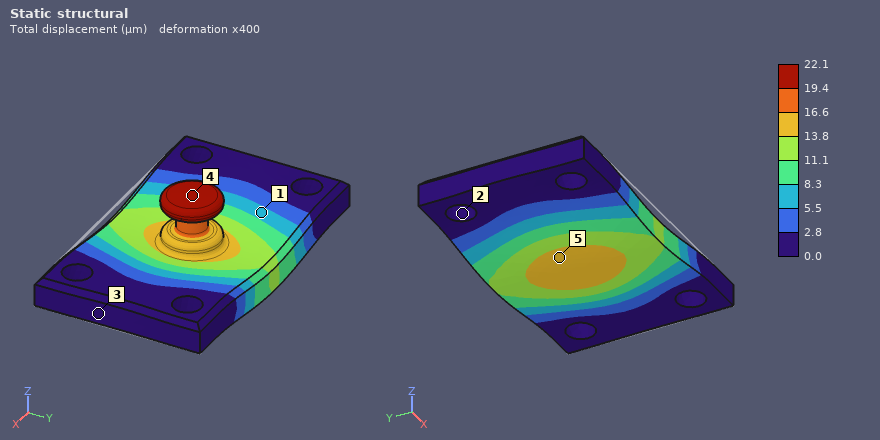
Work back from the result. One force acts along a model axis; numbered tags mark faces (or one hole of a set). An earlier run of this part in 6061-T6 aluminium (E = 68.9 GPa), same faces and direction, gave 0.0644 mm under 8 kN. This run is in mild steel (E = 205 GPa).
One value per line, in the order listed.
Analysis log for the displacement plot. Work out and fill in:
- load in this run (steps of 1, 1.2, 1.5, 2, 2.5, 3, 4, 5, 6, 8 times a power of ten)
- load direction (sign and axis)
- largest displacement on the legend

8 kN
-Z
22.1 µm
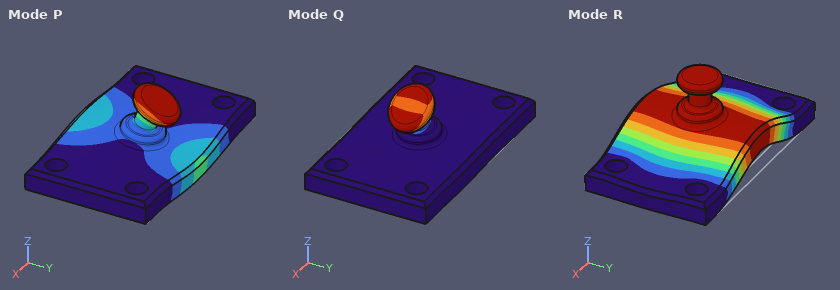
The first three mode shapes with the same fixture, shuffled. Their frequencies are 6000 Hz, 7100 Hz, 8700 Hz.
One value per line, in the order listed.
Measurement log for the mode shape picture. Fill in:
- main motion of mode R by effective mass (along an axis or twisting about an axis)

along Z
